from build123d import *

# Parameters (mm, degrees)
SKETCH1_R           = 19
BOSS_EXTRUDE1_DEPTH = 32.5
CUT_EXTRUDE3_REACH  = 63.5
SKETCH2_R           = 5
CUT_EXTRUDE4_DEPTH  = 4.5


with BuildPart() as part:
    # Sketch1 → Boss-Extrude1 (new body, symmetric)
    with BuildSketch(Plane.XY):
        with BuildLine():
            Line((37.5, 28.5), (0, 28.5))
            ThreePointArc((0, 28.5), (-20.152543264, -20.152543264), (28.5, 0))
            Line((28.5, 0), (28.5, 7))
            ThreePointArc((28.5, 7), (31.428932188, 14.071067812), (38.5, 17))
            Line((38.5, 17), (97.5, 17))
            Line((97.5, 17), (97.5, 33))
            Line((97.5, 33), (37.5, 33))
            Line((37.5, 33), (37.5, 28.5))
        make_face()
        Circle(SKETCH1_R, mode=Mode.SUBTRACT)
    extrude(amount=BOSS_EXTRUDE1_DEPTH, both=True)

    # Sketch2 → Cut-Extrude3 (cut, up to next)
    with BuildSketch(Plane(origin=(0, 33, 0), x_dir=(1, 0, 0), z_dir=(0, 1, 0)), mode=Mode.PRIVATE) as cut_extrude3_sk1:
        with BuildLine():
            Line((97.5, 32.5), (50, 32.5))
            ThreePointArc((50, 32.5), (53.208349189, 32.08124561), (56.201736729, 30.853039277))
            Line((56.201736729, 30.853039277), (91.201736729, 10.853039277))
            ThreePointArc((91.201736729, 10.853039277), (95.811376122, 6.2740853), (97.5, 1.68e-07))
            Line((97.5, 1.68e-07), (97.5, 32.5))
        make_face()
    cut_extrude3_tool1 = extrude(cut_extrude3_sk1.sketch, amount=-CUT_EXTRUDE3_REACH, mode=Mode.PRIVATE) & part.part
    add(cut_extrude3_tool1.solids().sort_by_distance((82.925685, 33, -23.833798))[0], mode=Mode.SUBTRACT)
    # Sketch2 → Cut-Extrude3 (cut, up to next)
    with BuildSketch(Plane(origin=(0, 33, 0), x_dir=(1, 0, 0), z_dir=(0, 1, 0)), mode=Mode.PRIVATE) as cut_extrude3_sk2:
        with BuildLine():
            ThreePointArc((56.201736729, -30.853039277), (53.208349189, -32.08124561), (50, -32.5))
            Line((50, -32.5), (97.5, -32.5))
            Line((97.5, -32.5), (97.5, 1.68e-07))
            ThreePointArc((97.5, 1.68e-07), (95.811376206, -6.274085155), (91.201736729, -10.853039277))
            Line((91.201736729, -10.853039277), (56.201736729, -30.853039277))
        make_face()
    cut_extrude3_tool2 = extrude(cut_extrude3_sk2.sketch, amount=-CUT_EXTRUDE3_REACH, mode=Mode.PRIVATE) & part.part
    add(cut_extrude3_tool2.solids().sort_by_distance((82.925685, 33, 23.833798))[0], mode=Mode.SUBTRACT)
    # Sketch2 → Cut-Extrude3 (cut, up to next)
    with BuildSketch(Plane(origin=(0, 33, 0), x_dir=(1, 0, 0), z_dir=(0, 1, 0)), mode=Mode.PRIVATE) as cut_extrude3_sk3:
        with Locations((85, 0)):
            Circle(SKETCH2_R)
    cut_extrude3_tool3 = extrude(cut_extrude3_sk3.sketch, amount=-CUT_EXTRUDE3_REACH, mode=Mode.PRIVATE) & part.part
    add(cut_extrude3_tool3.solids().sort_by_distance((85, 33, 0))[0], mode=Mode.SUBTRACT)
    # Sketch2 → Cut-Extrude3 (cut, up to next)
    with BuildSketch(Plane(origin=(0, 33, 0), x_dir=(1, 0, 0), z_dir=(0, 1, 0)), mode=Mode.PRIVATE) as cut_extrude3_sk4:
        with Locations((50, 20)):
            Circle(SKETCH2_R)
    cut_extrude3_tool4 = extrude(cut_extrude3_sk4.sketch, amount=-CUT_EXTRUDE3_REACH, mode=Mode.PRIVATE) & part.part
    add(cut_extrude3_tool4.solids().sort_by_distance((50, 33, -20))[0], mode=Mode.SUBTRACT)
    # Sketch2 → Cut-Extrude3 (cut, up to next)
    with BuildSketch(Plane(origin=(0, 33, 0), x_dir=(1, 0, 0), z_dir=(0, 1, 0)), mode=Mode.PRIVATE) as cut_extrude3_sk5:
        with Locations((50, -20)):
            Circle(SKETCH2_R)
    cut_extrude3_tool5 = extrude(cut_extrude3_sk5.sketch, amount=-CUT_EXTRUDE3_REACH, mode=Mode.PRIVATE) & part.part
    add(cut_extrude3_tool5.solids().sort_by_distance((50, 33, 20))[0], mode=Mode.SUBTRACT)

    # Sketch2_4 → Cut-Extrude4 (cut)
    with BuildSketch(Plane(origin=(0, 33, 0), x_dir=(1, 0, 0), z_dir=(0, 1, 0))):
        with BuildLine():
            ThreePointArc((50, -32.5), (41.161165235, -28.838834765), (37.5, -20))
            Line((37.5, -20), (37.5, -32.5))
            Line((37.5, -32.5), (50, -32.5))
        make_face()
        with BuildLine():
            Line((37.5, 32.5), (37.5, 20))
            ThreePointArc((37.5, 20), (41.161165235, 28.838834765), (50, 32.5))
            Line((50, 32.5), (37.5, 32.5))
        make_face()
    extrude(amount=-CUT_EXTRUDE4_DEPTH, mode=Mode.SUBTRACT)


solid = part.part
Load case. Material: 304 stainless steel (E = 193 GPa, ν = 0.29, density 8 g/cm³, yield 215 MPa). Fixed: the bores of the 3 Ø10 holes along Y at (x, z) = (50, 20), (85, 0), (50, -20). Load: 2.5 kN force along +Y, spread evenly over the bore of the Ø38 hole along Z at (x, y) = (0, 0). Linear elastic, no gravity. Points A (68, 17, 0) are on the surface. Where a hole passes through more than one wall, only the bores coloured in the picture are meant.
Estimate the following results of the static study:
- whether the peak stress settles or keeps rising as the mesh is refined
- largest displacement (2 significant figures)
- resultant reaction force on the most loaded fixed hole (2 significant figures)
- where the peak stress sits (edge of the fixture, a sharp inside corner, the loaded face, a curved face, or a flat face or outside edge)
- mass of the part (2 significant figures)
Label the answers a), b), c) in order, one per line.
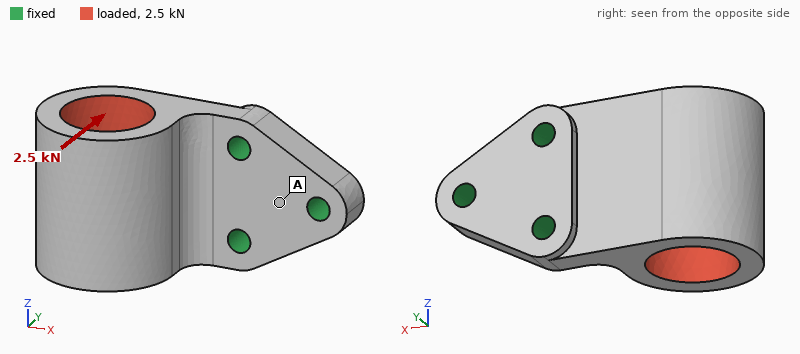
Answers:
a) keeps rising
b) 74 µm
c) 1.5 kN
d) edge of the fixture
e) 1.2 kg
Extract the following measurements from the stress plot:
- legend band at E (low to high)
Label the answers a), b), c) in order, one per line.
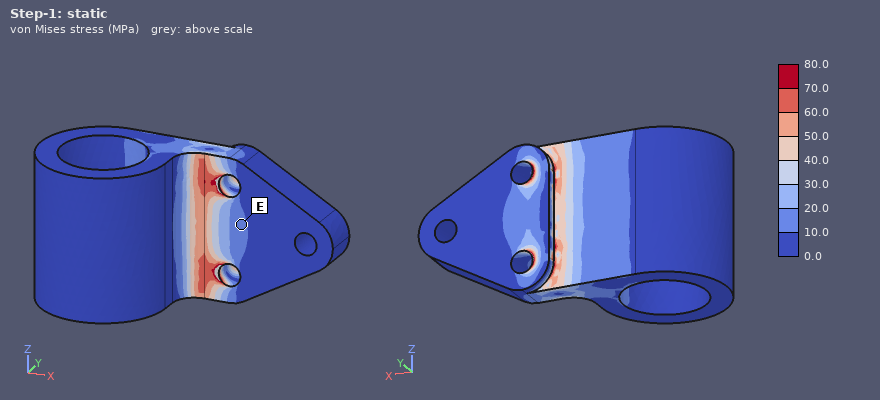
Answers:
a) 10.0 to 20.0 MPa
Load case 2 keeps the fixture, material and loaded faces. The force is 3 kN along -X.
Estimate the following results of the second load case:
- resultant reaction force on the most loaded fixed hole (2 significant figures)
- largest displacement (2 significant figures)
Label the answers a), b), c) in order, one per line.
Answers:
a) 1.4 kN
b) 57 µm
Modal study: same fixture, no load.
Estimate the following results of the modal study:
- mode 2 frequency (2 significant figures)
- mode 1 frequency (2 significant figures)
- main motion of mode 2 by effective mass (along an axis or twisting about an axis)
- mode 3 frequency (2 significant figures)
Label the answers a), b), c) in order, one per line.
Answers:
a) 3200 Hz
b) 1100 Hz
c) along Z
d) 5100 Hz
